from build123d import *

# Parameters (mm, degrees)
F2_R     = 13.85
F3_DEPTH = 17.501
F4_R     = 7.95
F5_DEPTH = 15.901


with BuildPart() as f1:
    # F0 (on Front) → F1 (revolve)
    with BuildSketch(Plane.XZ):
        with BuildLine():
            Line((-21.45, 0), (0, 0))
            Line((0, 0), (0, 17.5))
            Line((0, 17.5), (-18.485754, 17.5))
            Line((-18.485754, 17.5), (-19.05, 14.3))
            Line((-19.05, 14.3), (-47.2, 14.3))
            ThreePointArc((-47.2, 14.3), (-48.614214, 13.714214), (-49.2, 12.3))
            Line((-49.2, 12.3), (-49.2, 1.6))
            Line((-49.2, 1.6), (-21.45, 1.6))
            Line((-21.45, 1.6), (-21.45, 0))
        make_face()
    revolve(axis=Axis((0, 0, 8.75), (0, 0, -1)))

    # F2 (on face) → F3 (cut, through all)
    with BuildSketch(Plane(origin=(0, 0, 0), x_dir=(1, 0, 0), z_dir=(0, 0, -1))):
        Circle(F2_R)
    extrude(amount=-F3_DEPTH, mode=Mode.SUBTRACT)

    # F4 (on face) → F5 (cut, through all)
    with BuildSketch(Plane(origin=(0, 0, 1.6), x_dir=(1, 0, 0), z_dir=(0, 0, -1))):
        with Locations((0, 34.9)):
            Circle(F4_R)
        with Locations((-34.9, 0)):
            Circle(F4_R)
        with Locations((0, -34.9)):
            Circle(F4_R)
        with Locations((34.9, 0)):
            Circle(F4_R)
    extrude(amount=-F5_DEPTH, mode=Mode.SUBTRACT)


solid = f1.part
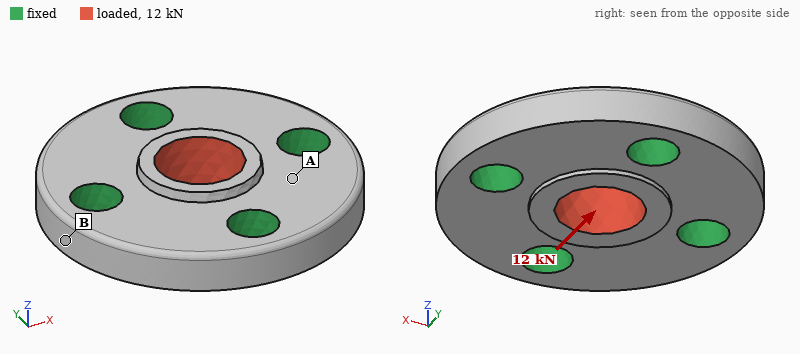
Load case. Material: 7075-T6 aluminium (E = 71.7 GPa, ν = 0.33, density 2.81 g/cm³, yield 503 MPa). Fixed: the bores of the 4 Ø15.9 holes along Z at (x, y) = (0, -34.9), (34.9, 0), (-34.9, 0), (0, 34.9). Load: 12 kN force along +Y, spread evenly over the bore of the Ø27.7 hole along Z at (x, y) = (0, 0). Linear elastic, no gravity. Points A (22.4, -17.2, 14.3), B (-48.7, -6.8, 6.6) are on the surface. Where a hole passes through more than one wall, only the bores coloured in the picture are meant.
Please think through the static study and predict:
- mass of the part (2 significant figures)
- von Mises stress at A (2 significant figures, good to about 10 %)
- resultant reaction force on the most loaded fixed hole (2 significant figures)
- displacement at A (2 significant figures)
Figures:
230 g
4.2 MPa
3.9 kN
1.6 µm
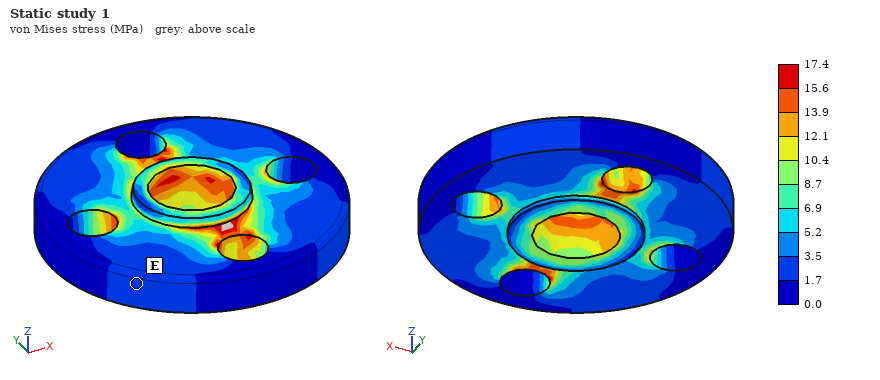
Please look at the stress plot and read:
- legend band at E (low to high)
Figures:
1.7 to 3.5 MPa
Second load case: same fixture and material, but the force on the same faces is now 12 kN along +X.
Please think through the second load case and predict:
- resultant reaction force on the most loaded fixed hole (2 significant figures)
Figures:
3.9 kN
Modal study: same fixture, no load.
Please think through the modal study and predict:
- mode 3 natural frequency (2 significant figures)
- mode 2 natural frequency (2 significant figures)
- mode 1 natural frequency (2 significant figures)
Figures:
19 kHz
19 kHz
19 kHz
